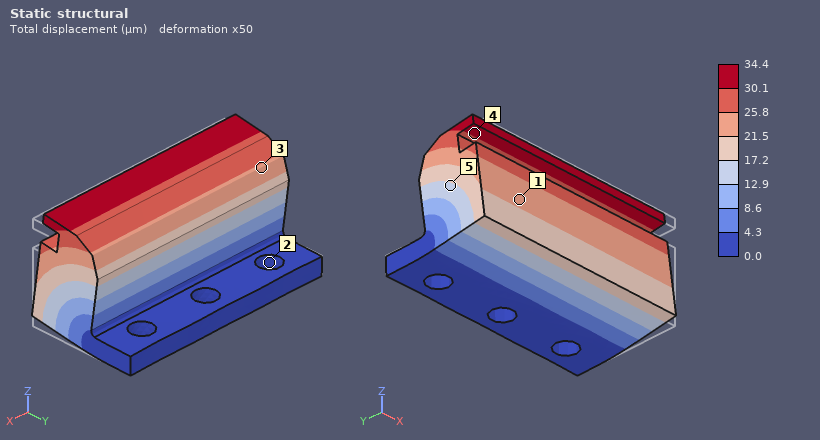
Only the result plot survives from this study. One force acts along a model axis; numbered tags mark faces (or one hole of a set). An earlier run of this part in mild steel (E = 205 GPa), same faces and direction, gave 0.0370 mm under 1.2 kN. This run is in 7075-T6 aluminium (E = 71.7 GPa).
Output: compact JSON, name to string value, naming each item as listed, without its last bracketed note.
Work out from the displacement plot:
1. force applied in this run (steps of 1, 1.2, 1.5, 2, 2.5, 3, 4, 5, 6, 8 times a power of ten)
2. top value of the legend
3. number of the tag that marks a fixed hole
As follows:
{"force applied in this run": "400 N", "top value of the legend": "34.4 µm", "number of the tag that marks a fixed hole": "2"}
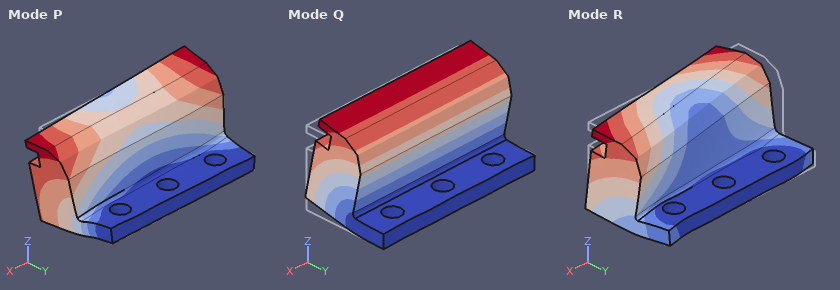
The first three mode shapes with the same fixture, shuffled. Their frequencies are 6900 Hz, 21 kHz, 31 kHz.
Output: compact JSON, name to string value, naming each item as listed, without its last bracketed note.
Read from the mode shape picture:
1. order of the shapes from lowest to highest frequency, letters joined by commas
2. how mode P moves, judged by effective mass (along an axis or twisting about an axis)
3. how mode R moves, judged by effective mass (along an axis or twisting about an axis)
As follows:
{"order of the shapes from lowest to highest frequency, letters joined by commas": "Q, P, R", "how mode P moves, judged by effective mass": "along X", "how mode R moves, judged by effective mass": "along X"}
